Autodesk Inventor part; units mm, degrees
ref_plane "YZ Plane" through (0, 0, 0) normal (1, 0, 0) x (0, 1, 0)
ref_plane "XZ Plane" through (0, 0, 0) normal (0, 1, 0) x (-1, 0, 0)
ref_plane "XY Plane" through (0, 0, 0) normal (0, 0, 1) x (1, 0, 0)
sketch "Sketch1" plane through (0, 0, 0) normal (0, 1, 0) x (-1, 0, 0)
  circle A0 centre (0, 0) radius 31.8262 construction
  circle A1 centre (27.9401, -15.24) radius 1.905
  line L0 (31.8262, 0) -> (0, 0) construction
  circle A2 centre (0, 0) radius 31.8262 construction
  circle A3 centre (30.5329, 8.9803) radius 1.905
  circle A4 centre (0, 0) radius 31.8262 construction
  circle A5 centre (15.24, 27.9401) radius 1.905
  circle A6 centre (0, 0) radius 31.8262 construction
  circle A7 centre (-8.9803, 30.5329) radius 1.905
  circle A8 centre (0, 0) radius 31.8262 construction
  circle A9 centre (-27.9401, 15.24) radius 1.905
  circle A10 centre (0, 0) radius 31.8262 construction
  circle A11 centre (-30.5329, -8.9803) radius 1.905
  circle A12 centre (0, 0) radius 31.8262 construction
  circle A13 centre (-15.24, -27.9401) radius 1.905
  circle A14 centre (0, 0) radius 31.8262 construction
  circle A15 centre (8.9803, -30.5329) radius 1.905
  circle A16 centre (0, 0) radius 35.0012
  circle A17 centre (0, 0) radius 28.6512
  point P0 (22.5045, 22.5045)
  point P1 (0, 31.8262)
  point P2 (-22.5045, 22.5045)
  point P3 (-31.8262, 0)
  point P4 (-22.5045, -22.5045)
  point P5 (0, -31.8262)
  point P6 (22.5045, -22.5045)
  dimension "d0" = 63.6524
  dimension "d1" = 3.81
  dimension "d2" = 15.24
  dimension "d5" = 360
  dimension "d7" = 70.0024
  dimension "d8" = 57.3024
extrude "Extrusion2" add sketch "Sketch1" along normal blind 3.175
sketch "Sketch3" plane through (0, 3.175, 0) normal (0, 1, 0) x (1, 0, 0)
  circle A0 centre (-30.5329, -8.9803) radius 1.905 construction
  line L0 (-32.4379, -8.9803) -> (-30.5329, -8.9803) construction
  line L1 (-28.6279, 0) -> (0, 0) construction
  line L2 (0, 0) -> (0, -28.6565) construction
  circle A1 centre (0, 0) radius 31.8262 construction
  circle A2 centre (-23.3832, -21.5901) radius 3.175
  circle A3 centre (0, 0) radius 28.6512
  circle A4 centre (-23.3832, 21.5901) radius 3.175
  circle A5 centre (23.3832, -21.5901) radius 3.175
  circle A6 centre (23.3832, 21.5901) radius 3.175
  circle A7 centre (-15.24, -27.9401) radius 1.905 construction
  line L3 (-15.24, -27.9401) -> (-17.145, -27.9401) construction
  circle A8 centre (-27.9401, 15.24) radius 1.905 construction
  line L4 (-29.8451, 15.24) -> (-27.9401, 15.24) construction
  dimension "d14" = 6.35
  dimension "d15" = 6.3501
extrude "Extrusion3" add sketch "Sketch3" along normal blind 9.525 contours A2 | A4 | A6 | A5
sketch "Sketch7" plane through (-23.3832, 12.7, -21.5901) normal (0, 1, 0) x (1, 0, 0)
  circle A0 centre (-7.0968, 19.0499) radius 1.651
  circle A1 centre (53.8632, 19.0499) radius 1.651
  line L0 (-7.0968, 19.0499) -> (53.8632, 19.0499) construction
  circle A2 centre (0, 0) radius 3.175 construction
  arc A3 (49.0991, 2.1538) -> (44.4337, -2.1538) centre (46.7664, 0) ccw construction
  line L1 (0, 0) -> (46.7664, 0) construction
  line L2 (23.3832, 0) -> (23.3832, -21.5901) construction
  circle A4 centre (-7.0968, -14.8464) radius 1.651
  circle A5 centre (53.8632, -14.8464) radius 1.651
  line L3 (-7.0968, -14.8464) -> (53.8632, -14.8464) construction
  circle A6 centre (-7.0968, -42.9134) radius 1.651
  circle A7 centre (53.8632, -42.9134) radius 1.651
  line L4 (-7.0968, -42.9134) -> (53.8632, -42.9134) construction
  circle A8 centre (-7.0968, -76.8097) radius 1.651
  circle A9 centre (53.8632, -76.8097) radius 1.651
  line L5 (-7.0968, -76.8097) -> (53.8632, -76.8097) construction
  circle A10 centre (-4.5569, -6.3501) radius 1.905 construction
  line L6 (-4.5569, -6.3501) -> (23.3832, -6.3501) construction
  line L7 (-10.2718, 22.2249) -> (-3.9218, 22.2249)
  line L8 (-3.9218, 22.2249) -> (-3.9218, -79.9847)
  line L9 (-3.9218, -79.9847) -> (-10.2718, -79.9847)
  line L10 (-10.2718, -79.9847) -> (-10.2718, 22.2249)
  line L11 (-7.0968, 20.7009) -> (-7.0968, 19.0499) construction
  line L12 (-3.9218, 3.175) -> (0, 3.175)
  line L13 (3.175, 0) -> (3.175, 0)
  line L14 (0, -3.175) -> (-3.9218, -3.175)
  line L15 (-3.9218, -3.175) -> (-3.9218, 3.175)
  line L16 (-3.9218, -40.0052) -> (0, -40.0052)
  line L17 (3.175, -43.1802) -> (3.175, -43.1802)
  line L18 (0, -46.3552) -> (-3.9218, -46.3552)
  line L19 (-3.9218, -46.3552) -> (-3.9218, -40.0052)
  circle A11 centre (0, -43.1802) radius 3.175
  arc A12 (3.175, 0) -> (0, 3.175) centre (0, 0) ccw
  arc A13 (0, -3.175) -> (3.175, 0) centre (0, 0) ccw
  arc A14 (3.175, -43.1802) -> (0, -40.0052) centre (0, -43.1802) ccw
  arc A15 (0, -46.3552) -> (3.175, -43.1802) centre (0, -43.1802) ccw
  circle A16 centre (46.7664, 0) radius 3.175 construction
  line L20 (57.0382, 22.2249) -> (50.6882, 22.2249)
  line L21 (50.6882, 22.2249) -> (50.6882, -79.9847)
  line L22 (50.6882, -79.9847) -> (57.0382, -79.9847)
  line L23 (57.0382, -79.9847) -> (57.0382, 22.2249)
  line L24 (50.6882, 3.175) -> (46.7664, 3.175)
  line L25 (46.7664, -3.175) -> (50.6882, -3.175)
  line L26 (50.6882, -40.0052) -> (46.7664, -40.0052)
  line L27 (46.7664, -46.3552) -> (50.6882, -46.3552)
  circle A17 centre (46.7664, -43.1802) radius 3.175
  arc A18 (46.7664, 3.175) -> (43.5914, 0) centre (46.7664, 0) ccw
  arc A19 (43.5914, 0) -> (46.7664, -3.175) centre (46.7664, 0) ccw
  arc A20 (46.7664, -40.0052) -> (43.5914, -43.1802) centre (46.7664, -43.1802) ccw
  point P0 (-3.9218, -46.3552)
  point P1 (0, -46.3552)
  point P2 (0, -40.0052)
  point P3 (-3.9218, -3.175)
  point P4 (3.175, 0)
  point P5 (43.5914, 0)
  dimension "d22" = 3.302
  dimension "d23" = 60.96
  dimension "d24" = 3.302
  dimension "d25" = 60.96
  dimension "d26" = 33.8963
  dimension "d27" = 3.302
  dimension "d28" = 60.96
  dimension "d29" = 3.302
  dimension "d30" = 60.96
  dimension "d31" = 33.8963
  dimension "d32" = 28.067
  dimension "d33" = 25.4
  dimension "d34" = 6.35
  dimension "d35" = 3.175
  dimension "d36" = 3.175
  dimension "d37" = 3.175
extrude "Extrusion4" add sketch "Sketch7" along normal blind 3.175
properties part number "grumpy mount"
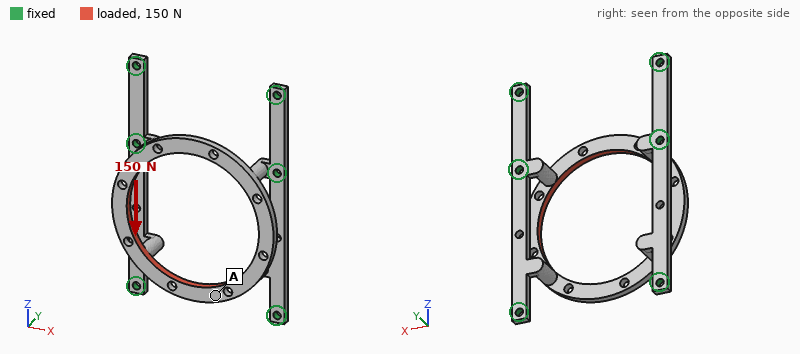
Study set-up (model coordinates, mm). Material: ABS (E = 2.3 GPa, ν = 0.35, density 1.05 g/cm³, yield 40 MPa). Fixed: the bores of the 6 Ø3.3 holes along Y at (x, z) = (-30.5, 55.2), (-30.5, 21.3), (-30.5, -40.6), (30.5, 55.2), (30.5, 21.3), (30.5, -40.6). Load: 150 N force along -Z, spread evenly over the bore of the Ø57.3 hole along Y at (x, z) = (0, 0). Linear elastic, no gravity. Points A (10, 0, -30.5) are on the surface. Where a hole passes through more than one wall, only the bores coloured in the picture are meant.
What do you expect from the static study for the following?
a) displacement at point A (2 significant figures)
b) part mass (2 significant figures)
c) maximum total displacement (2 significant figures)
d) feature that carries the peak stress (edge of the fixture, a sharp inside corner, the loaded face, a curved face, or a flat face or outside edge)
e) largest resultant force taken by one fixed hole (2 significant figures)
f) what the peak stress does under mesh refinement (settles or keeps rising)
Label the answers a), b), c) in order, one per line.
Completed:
a) 0.79 mm
b) 9.8 g
c) 0.90 mm
d) edge of the fixture
e) 50 N
f) keeps rising
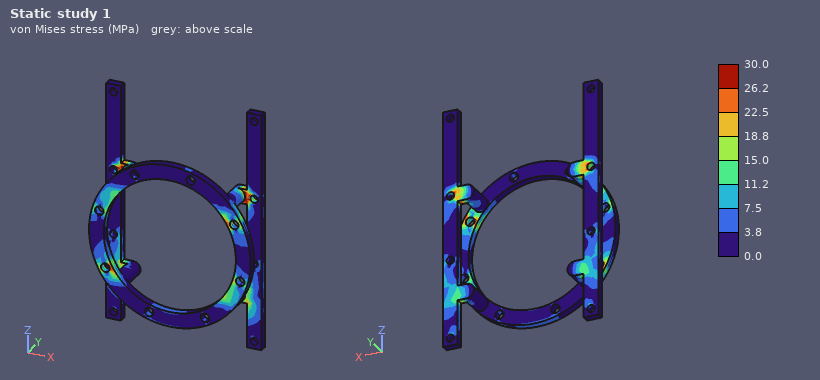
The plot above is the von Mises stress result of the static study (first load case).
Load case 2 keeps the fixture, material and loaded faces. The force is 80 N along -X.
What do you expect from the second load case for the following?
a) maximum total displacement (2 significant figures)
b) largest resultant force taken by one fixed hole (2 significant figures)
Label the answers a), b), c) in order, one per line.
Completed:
a) 0.53 mm
b) 27 N
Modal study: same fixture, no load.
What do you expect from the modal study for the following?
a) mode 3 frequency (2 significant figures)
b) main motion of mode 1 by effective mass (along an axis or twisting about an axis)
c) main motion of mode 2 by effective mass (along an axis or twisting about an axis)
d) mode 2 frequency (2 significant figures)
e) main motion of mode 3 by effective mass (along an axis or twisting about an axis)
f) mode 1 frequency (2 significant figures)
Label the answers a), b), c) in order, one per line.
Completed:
a) 1000 Hz
b) along Y
c) along X
d) 970 Hz
e) twisting about Z
f) 890 Hz
